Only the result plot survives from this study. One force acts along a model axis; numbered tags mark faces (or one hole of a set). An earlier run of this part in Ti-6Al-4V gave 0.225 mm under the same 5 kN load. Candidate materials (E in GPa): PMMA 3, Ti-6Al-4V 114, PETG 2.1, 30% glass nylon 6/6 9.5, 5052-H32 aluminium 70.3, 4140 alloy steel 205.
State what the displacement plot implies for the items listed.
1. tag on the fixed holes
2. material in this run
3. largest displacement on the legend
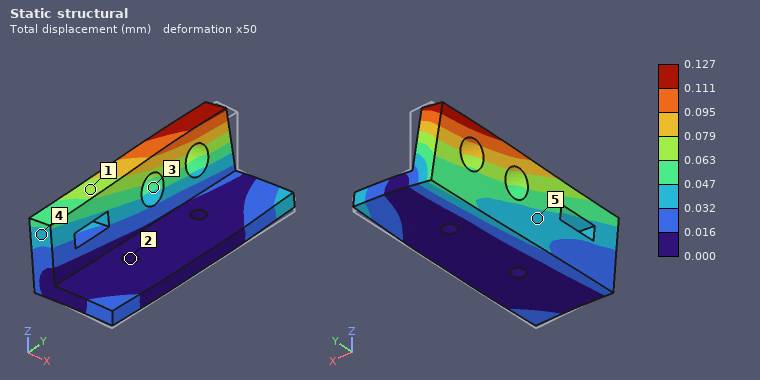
2
4140 alloy steel
0.127 mm
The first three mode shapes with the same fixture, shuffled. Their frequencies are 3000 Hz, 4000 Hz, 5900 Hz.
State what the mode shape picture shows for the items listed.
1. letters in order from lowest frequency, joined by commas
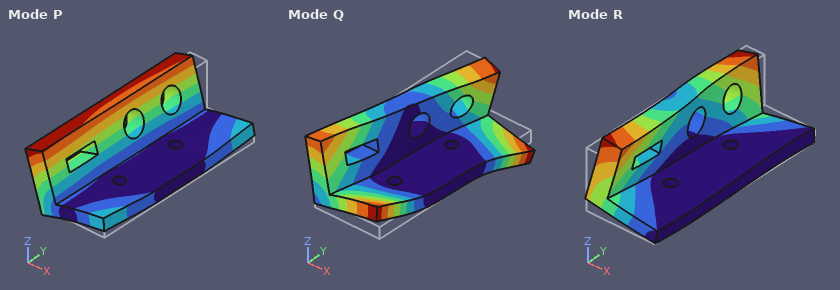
P, R, Q
